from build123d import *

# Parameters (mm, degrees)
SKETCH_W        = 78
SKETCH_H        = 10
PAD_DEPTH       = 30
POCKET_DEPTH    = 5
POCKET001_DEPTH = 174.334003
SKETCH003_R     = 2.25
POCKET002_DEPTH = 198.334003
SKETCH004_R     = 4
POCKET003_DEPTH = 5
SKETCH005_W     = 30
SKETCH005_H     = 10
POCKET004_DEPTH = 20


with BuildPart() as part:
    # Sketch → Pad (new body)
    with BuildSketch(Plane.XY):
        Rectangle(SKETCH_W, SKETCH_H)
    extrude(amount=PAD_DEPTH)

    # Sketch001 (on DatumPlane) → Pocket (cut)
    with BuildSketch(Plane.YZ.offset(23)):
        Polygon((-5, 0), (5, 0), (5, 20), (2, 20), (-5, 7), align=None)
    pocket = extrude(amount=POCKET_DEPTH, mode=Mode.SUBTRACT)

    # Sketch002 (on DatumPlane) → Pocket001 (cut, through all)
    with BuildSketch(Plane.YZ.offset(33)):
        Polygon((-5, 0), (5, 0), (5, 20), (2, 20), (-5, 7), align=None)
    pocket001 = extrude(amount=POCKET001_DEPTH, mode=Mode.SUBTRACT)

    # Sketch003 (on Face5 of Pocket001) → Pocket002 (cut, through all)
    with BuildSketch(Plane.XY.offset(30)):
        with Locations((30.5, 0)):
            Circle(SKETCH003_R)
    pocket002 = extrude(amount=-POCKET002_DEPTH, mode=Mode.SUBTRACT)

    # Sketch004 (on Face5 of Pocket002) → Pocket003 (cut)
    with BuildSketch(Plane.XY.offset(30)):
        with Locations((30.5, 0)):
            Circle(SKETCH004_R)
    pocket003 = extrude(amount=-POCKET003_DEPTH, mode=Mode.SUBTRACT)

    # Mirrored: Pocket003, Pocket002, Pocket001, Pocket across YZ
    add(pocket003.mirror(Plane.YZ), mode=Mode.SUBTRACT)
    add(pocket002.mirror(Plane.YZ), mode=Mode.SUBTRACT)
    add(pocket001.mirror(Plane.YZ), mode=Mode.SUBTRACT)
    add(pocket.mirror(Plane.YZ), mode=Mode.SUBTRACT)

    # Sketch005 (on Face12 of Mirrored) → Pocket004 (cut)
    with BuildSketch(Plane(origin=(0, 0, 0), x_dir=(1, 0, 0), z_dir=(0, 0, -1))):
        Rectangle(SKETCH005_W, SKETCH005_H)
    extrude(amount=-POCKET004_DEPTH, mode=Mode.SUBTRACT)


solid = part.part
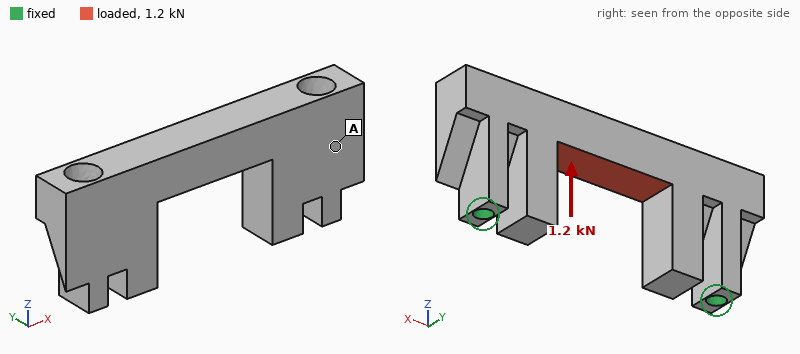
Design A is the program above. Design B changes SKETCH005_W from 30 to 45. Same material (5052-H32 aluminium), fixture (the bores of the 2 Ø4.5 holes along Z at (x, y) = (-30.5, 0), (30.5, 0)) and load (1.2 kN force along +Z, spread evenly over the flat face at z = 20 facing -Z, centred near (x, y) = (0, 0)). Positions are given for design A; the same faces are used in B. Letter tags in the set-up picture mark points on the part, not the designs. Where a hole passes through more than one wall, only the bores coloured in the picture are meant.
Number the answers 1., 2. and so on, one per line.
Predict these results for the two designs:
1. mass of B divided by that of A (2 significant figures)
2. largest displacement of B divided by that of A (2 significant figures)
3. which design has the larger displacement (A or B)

1. 0.76
2. 1.2
3. B
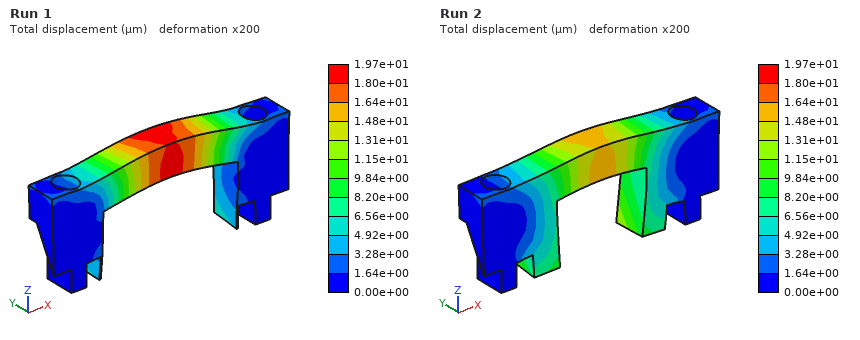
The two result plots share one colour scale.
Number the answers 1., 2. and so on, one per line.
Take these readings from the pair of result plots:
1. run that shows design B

1. Run 1
